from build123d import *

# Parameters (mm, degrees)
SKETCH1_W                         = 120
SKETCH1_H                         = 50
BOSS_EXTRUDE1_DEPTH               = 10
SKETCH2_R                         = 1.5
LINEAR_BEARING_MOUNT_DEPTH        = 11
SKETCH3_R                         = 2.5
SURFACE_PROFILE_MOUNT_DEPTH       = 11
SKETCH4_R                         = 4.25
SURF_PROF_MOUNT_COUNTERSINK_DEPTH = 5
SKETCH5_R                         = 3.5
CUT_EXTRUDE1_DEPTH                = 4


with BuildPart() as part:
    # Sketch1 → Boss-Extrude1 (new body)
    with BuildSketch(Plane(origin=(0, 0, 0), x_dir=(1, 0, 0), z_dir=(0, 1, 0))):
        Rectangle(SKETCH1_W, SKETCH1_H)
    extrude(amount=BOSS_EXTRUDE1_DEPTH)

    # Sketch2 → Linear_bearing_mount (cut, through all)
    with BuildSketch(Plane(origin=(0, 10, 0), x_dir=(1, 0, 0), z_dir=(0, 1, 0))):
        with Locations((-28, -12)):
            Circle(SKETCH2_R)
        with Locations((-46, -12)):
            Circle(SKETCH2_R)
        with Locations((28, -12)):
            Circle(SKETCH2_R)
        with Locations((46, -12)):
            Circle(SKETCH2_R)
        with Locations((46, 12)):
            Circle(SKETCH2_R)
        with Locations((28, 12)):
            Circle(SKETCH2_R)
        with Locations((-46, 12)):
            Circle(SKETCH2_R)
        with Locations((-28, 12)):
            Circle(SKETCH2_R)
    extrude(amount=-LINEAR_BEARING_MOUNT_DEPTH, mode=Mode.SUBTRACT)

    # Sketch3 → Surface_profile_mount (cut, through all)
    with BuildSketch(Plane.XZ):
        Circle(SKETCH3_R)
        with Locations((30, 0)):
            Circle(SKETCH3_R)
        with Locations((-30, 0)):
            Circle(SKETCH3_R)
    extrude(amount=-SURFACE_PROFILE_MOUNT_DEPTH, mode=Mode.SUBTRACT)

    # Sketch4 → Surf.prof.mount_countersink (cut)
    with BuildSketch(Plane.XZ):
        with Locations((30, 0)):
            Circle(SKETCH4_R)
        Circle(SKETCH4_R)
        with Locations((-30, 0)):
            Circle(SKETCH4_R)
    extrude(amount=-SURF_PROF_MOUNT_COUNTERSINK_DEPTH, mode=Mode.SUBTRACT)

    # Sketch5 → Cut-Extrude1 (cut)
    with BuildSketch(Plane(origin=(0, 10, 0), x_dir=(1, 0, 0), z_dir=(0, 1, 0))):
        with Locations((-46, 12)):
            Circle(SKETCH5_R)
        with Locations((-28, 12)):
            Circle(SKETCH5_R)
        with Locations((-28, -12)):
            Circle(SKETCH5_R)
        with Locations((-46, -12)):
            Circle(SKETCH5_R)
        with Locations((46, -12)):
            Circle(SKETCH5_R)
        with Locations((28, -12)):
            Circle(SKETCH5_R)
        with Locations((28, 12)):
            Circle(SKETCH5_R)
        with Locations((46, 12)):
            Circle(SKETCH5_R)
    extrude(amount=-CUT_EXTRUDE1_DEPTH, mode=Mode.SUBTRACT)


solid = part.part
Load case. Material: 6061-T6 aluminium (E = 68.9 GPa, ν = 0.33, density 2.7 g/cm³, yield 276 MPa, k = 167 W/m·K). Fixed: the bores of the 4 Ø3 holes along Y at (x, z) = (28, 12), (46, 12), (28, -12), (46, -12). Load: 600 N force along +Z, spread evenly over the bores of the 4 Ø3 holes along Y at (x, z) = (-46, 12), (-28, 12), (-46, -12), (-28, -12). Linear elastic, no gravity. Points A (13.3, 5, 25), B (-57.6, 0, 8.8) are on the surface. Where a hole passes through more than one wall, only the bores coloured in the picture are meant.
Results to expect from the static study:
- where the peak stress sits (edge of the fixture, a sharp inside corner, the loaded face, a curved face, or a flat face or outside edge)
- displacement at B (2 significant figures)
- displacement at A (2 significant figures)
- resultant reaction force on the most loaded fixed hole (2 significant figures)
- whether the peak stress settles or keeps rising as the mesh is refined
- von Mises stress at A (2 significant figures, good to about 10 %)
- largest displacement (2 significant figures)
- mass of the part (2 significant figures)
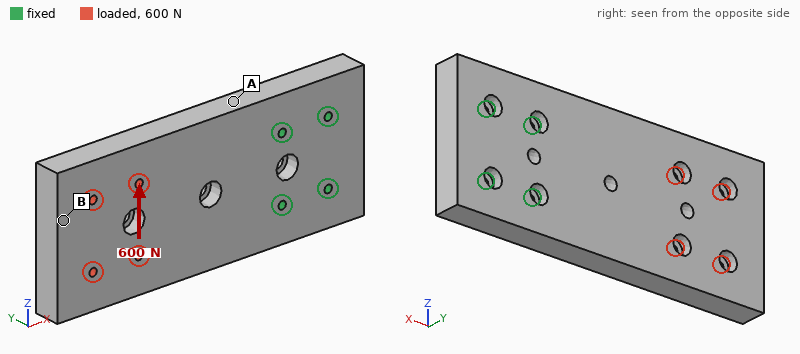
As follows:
edge of the fixture
24 µm
5.4 µm
970 N
keeps rising
7.2 MPa
26 µm
150 g
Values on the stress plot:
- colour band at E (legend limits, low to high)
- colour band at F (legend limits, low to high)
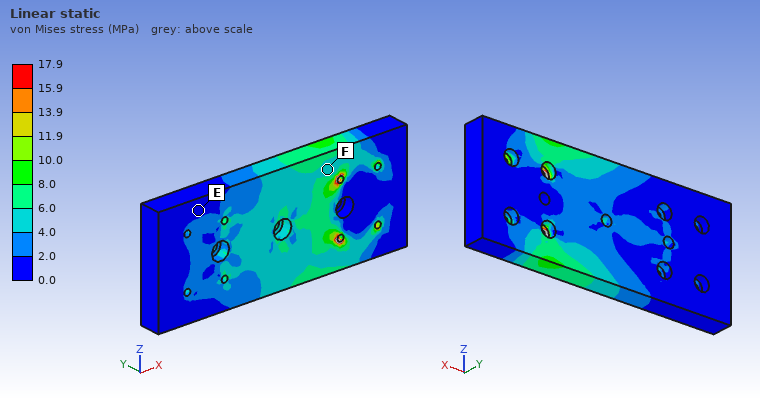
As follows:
0.0 to 2.0 MPa
4.0 to 6.0 MPa
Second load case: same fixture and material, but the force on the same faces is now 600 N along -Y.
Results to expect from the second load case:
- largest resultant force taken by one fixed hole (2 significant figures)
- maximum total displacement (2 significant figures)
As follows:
1.2 kN
0.40 mm
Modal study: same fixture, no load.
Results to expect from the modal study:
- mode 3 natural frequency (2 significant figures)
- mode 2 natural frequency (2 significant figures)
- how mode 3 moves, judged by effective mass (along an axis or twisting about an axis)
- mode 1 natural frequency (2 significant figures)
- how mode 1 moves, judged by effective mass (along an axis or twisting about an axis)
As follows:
3600 Hz
3300 Hz
along Z
920 Hz
along Y
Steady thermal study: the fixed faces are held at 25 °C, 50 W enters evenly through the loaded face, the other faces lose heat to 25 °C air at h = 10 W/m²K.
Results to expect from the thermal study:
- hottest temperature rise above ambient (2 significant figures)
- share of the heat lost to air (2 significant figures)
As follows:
45 K
6.8 %
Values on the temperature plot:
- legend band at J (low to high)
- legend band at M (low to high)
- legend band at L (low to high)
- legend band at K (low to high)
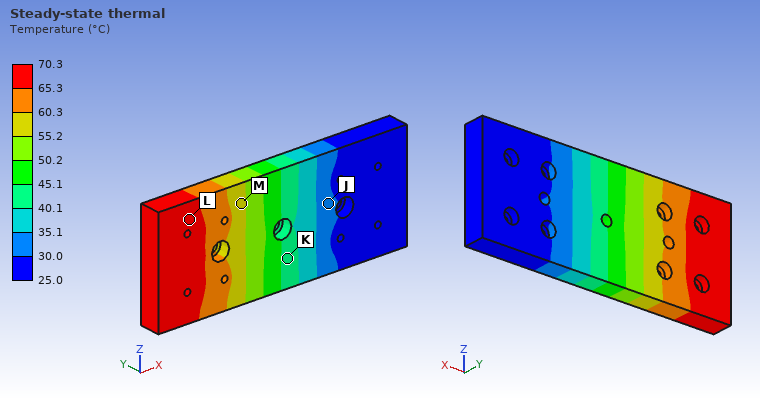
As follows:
30.0 to 35.1 °C
55.2 to 60.3 °C
65.3 to 70.3 °C
40.1 to 45.1 °C
